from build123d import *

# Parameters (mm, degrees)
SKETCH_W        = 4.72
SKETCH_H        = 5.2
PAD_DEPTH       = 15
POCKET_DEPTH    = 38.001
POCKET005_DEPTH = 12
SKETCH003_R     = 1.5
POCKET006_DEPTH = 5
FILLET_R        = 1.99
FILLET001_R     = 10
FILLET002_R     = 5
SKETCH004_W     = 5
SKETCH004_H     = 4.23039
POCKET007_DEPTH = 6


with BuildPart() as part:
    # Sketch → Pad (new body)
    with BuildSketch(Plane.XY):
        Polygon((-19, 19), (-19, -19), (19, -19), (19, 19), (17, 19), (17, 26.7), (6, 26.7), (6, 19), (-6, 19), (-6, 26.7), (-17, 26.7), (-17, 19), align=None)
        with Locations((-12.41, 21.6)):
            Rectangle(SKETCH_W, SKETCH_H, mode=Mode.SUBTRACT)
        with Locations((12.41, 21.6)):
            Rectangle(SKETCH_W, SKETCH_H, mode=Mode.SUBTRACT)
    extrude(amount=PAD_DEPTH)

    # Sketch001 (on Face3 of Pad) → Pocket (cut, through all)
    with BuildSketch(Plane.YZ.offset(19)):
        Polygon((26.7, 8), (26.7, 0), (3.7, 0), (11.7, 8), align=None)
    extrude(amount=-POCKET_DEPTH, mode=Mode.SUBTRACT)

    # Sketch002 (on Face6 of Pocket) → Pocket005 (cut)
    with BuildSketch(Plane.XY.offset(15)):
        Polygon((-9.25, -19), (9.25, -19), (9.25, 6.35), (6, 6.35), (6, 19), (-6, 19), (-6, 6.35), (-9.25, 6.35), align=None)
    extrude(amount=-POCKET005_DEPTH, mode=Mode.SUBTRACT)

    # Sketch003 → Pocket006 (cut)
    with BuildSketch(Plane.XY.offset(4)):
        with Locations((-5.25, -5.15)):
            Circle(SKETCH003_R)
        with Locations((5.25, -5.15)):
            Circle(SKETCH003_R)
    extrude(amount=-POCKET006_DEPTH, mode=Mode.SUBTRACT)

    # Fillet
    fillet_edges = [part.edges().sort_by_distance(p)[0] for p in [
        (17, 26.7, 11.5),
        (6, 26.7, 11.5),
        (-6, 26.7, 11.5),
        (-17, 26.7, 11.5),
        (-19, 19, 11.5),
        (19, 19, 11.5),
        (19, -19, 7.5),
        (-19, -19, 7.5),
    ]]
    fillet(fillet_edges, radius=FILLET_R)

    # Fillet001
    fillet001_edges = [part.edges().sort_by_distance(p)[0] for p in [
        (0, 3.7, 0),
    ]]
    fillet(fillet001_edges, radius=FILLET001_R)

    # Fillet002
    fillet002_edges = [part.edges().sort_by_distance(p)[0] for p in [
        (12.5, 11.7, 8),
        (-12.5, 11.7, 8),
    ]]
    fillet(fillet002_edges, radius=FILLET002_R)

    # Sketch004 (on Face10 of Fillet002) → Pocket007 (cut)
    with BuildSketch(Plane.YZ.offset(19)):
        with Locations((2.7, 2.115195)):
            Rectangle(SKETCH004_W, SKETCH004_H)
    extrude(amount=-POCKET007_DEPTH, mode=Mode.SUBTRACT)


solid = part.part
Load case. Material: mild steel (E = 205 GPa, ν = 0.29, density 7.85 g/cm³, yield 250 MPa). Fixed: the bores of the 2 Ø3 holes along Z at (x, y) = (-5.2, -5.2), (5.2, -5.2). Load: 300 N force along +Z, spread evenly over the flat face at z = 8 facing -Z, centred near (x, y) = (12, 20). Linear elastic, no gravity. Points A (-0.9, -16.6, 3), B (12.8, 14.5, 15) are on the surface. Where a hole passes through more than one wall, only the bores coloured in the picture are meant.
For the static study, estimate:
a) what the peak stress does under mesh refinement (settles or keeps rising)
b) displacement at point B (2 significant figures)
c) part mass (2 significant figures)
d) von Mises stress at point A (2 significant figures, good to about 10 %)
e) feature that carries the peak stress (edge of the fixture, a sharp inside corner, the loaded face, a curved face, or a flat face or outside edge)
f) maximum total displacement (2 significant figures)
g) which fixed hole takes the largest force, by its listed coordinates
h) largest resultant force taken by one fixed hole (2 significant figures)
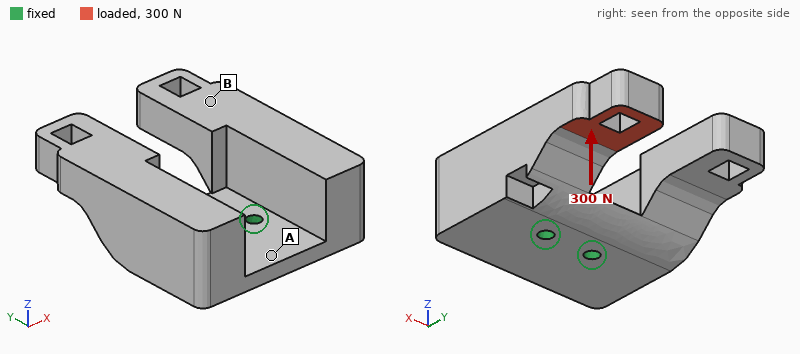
keeps rising
58 µm
94 g
43 MPa
edge of the fixture
87 µm
(5.2, -5.2)
370 N
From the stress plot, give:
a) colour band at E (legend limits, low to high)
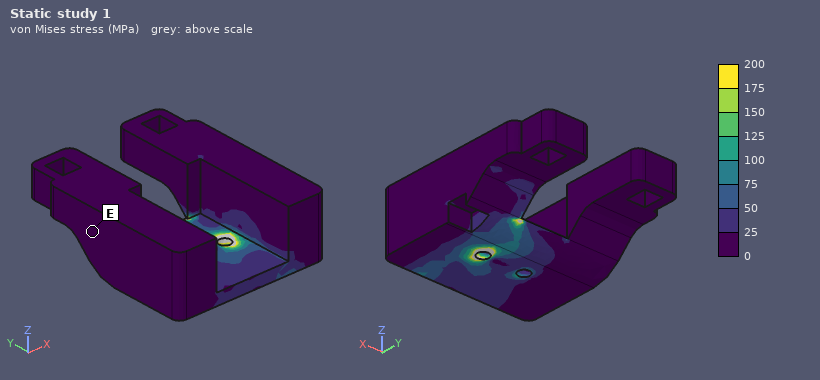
0 to 25 MPa
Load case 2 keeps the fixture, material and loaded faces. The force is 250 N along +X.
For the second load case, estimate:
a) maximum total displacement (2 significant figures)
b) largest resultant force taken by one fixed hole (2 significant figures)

29 µm
490 N
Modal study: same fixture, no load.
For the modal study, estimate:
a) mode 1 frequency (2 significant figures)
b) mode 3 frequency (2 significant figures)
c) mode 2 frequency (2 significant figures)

2600 Hz
3100 Hz
3000 Hz
